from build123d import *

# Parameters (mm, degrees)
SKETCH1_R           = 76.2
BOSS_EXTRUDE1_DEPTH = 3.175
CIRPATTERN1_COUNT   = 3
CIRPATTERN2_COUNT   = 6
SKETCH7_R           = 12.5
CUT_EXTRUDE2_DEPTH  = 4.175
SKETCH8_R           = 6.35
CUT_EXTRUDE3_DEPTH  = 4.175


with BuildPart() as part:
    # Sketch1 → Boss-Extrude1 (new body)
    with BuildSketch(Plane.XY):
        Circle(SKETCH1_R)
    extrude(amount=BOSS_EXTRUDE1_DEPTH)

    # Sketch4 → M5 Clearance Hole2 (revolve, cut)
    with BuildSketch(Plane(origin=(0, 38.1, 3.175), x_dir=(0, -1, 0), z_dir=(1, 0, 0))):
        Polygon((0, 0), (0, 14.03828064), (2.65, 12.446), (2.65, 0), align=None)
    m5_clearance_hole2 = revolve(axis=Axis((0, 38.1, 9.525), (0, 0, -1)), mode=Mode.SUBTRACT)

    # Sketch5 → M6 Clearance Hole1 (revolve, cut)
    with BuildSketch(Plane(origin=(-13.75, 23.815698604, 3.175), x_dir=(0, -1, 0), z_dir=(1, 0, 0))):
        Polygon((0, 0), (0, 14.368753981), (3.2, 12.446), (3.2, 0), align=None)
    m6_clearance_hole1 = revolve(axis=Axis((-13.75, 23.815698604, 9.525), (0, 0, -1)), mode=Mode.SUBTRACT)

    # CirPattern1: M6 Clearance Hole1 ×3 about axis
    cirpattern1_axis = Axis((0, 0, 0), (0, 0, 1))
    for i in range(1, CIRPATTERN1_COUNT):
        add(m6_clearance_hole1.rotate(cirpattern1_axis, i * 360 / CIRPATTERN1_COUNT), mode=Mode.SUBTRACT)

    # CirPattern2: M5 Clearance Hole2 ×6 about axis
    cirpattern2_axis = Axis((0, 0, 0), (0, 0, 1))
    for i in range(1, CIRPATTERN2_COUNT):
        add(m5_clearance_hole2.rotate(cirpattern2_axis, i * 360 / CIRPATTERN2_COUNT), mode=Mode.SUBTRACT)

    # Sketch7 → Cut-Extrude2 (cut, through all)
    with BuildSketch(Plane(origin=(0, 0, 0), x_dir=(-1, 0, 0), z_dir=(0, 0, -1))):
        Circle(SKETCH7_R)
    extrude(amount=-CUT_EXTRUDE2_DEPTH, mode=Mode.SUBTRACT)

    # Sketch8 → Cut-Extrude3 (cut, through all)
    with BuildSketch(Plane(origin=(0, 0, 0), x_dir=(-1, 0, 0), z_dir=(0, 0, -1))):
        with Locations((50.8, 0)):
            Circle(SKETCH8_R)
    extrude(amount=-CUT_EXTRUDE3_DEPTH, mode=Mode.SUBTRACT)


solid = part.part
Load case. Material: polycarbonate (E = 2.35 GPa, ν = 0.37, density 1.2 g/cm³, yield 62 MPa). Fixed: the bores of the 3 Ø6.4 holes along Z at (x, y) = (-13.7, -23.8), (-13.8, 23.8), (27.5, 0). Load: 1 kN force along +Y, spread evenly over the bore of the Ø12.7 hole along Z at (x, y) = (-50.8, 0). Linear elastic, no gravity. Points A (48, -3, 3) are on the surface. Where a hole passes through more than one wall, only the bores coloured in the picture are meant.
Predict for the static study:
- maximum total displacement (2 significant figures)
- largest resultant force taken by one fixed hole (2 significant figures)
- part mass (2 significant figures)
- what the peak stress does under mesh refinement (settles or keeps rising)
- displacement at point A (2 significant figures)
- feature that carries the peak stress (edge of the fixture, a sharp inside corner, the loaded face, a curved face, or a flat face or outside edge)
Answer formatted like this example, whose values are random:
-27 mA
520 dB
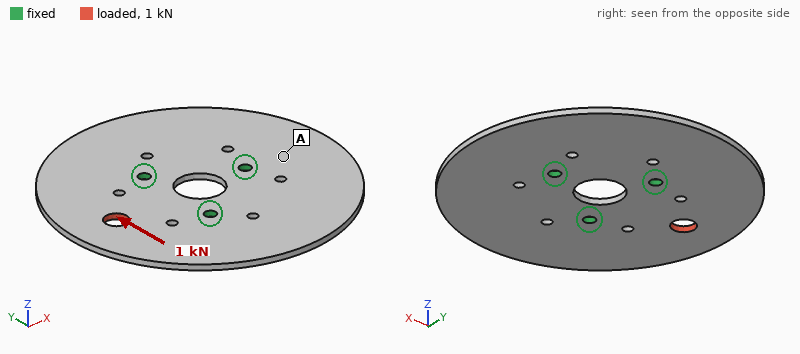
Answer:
0.30 mm
800 N
66 g
keeps rising
0.056 mm
edge of the fixture
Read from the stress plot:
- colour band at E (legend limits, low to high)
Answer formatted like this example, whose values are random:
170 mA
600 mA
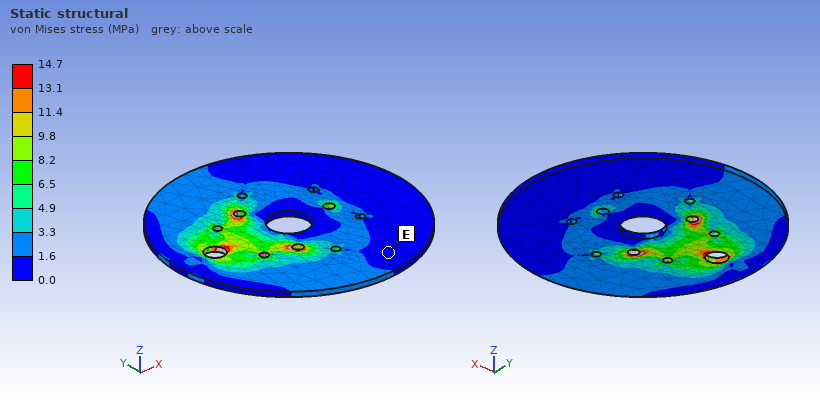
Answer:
0.0 to 1.6 MPa
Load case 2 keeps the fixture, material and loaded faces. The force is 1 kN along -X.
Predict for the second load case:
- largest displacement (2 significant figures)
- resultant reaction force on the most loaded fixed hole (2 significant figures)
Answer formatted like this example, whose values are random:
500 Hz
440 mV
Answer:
0.17 mm
500 N
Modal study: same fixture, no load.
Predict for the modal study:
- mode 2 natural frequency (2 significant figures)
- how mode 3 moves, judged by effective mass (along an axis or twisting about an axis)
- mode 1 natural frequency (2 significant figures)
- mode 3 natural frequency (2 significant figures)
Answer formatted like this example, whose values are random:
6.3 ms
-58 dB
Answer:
220 Hz
along Z
210 Hz
250 Hz
